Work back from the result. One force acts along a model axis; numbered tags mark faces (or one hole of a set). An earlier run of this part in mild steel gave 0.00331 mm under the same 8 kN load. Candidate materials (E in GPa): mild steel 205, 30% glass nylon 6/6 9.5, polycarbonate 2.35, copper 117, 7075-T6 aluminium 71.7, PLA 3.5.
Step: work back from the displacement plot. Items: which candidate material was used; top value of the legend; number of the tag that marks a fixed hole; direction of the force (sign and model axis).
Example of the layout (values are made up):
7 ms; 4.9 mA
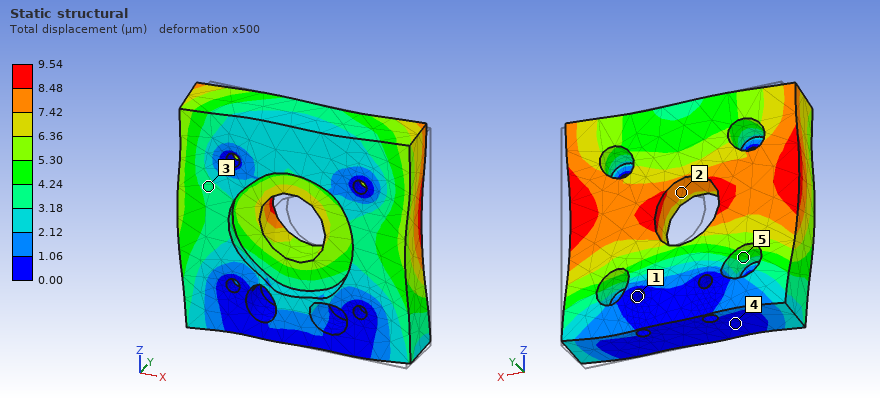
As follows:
7075-T6 aluminium; 9.54 µm; 1; -X
